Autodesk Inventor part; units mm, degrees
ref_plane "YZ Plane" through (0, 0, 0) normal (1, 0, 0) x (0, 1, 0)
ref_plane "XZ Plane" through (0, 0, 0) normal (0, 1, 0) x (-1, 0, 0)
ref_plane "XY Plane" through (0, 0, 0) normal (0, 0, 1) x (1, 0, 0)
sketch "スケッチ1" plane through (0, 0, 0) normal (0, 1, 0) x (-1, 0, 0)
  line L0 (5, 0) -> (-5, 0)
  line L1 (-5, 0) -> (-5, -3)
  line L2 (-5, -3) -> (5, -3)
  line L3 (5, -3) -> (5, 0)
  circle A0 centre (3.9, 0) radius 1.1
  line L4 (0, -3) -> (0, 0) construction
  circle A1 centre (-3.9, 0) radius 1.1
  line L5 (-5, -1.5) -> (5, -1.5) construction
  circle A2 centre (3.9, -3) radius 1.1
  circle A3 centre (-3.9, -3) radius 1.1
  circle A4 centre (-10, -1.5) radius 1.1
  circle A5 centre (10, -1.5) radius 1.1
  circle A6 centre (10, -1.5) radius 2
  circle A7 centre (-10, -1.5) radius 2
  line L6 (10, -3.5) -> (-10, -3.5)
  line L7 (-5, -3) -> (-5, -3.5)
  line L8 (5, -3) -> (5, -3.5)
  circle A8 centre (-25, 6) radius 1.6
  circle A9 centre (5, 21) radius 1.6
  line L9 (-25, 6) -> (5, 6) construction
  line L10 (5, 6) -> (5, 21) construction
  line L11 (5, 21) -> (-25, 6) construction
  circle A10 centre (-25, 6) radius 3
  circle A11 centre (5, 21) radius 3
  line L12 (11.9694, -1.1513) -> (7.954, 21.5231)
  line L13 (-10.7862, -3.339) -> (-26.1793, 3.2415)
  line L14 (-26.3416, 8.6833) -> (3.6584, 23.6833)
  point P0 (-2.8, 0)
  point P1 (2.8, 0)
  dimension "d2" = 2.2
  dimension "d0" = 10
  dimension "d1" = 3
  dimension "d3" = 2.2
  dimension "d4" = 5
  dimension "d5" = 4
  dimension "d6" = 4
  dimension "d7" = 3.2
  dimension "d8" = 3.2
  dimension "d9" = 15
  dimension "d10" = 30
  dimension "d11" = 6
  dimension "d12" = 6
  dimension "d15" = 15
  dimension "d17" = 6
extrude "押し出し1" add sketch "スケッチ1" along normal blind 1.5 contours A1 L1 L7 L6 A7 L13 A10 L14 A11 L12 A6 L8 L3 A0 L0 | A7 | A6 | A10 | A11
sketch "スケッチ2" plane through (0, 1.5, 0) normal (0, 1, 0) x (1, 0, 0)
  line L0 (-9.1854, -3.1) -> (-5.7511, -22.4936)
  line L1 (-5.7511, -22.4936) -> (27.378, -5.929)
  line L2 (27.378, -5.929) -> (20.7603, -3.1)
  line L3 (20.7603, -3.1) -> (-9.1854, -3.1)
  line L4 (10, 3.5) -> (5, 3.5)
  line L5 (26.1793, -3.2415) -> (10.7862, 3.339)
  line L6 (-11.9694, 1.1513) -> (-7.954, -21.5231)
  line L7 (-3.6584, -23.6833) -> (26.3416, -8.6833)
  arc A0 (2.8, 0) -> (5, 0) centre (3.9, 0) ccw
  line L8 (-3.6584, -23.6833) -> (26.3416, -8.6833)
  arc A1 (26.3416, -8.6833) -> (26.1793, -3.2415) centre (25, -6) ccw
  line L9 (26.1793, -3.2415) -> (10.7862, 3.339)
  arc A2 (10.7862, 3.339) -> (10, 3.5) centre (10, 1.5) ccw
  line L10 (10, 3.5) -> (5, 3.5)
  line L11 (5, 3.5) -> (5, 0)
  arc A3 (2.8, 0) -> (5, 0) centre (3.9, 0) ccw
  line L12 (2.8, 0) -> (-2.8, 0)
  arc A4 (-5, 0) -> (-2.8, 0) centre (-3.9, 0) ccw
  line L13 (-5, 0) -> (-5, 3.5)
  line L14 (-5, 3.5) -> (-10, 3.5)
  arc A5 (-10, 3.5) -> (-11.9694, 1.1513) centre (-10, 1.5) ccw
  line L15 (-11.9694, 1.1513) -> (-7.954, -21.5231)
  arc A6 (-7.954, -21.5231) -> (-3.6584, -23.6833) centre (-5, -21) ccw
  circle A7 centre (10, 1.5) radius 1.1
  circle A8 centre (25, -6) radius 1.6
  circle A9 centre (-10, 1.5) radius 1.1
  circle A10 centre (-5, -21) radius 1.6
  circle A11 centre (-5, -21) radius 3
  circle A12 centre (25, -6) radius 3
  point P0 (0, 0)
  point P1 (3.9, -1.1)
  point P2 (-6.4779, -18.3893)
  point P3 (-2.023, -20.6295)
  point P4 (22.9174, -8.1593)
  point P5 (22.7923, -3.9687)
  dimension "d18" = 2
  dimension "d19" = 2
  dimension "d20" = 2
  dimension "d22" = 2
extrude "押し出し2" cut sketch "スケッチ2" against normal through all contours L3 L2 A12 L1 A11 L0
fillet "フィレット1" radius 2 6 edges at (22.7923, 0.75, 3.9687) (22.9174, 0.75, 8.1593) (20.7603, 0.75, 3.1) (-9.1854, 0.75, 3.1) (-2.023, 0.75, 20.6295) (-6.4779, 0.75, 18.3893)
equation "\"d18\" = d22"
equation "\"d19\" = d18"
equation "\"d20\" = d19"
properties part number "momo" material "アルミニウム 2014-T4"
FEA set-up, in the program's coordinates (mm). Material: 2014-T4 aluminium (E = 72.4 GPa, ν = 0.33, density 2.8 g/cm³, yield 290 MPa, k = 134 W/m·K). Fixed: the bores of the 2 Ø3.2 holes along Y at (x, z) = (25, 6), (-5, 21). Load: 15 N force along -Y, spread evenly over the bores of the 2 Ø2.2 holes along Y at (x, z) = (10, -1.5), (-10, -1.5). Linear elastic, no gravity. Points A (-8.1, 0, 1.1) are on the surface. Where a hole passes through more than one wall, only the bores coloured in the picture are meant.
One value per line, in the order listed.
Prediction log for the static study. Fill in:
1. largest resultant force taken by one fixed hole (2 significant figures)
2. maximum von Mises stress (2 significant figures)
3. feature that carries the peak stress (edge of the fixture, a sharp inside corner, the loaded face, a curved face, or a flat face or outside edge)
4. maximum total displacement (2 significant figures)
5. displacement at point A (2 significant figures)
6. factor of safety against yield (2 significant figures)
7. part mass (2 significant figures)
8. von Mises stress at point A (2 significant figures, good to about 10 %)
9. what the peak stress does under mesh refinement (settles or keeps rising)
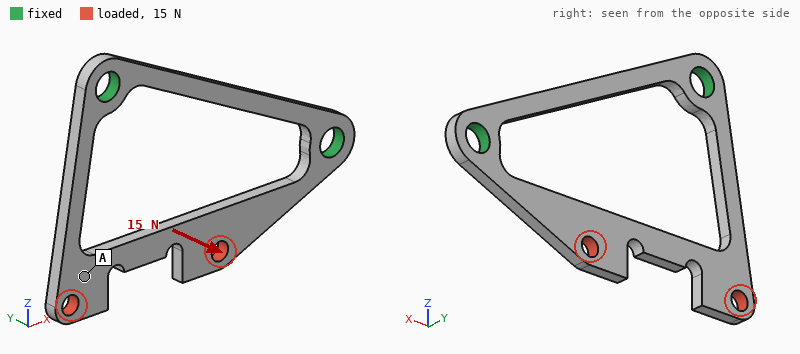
7.7 N
170 MPa
a curved face
0.45 mm
0.32 mm
1.7
1.2 g
18 MPa
settles
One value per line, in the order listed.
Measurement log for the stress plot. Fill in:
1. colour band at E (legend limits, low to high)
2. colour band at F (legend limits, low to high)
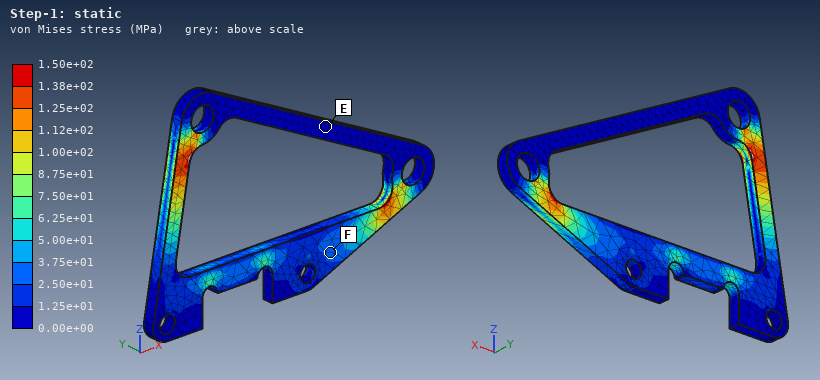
0.00e+00 to 1.25e+01 MPa
2.50e+01 to 3.75e+01 MPa
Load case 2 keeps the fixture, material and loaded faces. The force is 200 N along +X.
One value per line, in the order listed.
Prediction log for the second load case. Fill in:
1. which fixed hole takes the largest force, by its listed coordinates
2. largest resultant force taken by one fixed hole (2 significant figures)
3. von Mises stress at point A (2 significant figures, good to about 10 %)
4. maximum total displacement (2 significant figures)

(25, 6)
210 N
18 MPa
49 µm
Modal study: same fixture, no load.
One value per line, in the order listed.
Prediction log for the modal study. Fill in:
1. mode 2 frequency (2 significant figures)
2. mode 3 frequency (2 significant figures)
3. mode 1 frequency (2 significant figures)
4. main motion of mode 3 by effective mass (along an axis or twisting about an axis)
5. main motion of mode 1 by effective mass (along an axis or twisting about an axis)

4700 Hz
7500 Hz
1700 Hz
along Z
along Y
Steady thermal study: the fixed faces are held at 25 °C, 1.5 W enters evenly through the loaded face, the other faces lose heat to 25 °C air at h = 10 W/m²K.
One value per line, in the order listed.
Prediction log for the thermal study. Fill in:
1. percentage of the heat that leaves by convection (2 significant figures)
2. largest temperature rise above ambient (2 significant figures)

6.4 %
27 K
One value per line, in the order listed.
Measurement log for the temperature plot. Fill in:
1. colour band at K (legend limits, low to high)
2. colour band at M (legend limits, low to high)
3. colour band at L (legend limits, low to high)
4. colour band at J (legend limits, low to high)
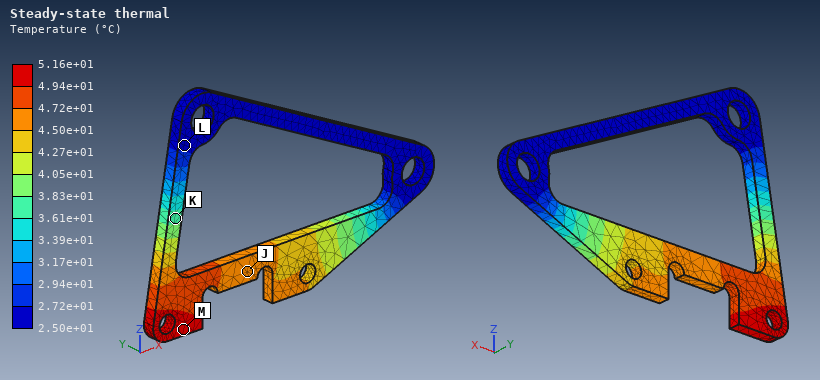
3.61e+01 to 3.83e+01 °C
4.94e+01 to 5.16e+01 °C
2.50e+01 to 2.72e+01 °C
4.50e+01 to 4.72e+01 °C
